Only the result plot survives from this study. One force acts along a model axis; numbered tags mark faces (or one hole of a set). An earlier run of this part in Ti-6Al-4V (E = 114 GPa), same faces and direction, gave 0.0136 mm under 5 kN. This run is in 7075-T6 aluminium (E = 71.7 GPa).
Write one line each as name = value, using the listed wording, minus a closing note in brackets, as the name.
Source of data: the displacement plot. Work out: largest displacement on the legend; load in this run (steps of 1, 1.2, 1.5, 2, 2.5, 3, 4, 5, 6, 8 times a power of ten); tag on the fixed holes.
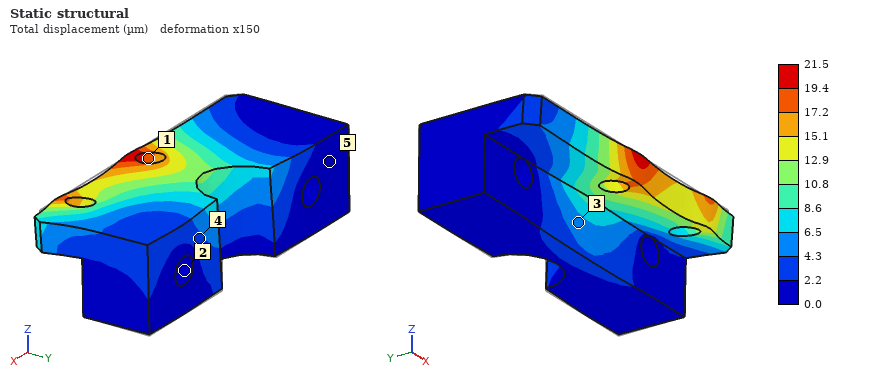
largest displacement on the legend = 21.5 µm
load in this run = 5 kN
tag on the fixed holes = 2
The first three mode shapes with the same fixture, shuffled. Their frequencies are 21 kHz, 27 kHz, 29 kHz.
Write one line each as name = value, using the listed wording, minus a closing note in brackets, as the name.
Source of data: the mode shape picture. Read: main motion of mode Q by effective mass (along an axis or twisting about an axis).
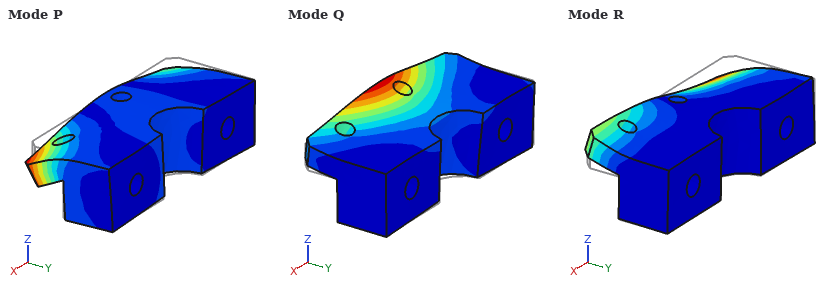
main motion of mode Q by effective mass = along Z
